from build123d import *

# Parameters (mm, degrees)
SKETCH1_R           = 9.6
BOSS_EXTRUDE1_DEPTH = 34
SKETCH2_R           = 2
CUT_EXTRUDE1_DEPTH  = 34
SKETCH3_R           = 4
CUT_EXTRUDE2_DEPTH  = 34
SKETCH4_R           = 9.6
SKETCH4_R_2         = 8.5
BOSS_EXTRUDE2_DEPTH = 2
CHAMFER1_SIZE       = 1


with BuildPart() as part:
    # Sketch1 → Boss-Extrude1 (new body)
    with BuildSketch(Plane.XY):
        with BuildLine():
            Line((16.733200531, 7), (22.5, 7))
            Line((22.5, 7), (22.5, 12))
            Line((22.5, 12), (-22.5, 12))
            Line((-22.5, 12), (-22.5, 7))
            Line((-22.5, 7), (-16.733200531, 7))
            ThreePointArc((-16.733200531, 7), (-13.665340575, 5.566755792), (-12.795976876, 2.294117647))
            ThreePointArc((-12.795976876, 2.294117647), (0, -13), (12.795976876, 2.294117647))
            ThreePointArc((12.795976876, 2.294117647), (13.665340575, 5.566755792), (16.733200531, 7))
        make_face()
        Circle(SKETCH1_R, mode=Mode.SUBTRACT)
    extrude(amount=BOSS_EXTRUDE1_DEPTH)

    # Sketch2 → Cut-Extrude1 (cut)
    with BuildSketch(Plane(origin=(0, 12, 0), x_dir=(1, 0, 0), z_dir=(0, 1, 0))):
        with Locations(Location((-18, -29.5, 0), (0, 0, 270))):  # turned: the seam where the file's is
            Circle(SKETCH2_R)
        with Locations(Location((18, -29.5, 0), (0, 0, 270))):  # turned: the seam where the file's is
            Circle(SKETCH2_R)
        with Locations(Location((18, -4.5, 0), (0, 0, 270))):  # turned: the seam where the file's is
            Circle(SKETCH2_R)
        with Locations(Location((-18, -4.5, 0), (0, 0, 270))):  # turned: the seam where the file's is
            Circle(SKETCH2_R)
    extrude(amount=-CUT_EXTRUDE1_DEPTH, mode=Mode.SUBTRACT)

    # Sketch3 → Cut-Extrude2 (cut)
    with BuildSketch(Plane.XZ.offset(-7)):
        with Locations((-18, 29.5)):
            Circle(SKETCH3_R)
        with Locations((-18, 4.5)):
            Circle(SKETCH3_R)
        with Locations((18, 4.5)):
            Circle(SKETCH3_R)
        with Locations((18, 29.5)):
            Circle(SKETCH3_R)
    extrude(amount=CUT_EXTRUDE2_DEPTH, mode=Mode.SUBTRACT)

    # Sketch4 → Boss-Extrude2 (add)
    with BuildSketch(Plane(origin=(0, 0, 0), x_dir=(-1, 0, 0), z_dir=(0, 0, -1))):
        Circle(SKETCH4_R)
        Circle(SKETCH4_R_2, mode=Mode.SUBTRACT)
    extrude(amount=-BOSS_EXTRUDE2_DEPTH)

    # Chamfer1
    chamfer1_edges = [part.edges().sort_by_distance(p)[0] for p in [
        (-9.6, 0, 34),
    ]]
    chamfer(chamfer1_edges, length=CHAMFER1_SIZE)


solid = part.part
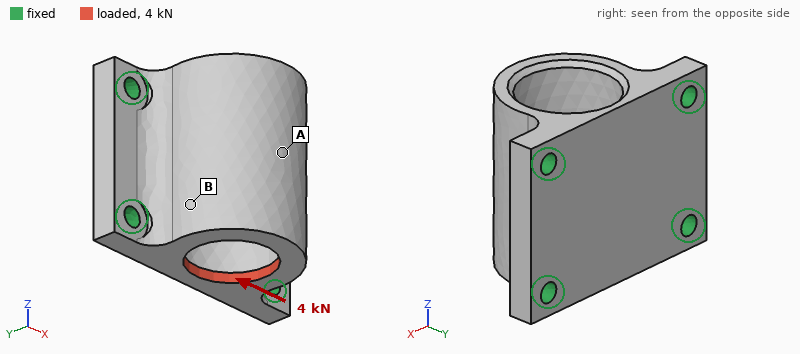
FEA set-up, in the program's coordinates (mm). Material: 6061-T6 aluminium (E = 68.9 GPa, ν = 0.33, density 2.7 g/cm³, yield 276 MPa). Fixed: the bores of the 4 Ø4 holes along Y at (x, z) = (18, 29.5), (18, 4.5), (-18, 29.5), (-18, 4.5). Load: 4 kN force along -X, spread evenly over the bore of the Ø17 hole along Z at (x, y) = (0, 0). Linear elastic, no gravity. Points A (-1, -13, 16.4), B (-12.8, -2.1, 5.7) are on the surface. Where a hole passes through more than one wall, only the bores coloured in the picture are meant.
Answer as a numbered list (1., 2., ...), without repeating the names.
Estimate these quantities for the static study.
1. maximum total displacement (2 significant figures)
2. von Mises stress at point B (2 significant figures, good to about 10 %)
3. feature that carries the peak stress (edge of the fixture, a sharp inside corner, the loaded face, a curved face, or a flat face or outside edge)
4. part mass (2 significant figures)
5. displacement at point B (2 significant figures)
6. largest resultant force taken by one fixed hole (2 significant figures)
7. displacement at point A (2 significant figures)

1. 72 µm
2. 44 MPa
3. the loaded face
4. 35 g
5. 36 µm
6. 1.6 kN
7. 29 µm
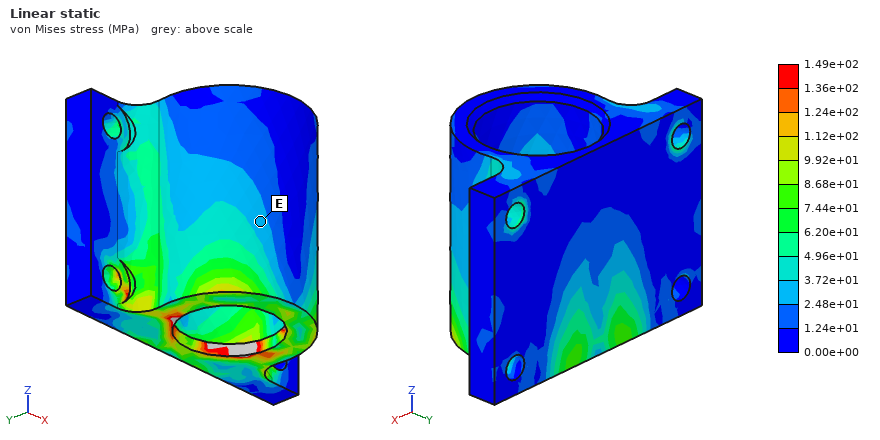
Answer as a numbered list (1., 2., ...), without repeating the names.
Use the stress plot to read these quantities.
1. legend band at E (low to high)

1. 2.48e+01 to 3.72e+01 MPa
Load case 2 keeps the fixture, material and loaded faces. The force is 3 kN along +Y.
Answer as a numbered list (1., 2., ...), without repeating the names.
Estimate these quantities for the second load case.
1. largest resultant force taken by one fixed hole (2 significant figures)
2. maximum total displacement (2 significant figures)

1. 1.7 kN
2. 44 µm
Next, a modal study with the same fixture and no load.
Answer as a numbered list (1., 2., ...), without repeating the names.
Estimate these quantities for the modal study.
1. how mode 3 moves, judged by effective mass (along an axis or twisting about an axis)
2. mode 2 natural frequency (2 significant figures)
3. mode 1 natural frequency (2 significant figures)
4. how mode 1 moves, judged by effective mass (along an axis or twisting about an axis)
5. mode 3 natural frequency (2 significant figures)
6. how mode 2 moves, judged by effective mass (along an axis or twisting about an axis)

1. along Y
2. 15 kHz
3. 12 kHz
4. along X
5. 17 kHz
6. along Z
